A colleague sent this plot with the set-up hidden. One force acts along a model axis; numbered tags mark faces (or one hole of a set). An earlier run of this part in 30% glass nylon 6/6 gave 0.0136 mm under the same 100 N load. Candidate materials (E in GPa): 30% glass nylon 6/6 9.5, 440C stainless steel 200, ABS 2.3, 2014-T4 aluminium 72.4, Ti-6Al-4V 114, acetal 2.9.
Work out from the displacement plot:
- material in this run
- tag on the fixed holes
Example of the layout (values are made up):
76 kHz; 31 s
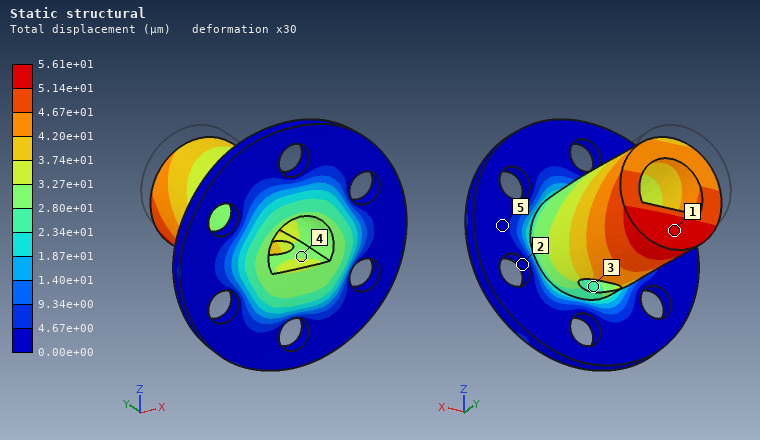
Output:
ABS; 2
